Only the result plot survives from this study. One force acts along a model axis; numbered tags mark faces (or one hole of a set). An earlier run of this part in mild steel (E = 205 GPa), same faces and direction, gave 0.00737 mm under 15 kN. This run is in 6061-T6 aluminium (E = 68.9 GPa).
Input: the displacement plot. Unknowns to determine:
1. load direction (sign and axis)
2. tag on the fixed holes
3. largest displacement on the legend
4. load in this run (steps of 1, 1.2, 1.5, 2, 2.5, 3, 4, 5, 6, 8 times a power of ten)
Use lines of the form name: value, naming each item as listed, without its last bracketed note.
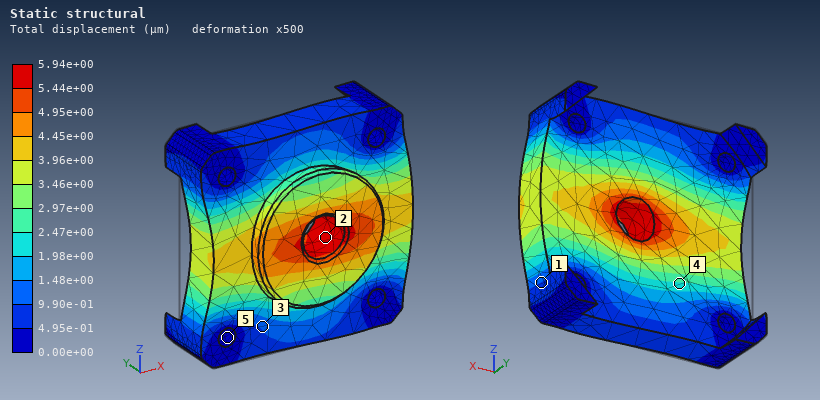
load direction: +X
tag on the fixed holes: 5
largest displacement on the legend: 5.94e+00 µm
load in this run: 4 kN
